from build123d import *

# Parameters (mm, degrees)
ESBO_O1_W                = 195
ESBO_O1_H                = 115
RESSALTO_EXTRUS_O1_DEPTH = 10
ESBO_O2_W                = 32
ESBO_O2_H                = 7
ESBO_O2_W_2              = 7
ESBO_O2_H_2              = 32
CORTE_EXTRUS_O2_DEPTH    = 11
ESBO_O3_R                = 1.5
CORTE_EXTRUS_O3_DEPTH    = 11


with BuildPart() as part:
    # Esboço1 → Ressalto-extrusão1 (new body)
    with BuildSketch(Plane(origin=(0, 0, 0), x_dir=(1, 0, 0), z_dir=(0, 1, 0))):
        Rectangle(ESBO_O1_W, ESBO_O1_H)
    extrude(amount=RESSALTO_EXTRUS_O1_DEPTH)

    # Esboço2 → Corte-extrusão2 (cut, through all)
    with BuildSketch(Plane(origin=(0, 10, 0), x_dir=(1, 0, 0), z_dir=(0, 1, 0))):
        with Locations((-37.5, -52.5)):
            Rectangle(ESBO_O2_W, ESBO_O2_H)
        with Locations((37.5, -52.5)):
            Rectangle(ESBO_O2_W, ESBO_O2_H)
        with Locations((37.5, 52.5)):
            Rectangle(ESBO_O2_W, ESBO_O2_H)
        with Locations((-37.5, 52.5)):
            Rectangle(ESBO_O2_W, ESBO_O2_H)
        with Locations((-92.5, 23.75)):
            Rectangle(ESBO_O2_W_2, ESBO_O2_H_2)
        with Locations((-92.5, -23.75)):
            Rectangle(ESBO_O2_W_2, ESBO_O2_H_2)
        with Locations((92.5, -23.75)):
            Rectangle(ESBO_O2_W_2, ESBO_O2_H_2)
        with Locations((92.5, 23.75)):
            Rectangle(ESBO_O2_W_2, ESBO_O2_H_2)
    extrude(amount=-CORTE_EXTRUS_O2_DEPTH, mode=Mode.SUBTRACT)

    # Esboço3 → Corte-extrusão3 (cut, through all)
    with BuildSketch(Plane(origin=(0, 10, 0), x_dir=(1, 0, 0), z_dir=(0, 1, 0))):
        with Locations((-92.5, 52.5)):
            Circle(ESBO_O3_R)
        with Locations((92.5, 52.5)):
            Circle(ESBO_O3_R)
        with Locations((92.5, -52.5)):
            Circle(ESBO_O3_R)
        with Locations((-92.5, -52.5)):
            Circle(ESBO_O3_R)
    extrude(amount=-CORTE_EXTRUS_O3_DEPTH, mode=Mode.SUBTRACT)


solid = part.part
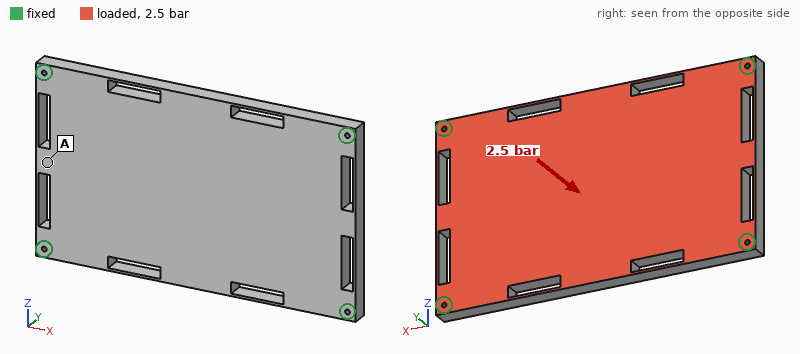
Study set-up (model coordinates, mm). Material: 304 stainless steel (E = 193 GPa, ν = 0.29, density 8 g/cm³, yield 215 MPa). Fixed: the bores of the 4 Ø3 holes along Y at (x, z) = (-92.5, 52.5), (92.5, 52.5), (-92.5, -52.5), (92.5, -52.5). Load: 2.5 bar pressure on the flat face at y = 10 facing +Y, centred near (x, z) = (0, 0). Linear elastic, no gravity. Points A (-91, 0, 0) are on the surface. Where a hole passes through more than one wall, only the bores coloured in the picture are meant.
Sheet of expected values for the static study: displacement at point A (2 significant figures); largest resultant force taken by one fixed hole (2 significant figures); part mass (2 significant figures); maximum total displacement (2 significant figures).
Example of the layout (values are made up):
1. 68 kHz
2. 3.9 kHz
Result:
1. 0.016 mm
2. 1.3 kN
3. 1.6 kg
4. 0.10 mm
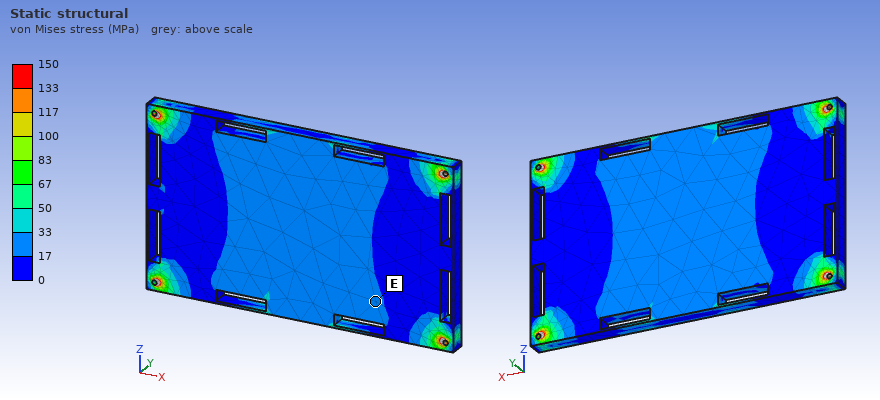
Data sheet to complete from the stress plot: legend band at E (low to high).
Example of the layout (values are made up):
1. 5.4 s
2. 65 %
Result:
1. 17 to 33 MPa
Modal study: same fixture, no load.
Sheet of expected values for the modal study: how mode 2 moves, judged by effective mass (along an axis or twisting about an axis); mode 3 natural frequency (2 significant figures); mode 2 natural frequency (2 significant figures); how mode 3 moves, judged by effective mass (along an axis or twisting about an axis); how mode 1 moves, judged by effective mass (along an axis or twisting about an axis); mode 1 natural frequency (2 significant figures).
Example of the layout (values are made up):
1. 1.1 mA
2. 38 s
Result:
1. twisting about X
2. 2700 Hz
3. 1900 Hz
4. twisting about Z
5. along Y
6. 1000 Hz
